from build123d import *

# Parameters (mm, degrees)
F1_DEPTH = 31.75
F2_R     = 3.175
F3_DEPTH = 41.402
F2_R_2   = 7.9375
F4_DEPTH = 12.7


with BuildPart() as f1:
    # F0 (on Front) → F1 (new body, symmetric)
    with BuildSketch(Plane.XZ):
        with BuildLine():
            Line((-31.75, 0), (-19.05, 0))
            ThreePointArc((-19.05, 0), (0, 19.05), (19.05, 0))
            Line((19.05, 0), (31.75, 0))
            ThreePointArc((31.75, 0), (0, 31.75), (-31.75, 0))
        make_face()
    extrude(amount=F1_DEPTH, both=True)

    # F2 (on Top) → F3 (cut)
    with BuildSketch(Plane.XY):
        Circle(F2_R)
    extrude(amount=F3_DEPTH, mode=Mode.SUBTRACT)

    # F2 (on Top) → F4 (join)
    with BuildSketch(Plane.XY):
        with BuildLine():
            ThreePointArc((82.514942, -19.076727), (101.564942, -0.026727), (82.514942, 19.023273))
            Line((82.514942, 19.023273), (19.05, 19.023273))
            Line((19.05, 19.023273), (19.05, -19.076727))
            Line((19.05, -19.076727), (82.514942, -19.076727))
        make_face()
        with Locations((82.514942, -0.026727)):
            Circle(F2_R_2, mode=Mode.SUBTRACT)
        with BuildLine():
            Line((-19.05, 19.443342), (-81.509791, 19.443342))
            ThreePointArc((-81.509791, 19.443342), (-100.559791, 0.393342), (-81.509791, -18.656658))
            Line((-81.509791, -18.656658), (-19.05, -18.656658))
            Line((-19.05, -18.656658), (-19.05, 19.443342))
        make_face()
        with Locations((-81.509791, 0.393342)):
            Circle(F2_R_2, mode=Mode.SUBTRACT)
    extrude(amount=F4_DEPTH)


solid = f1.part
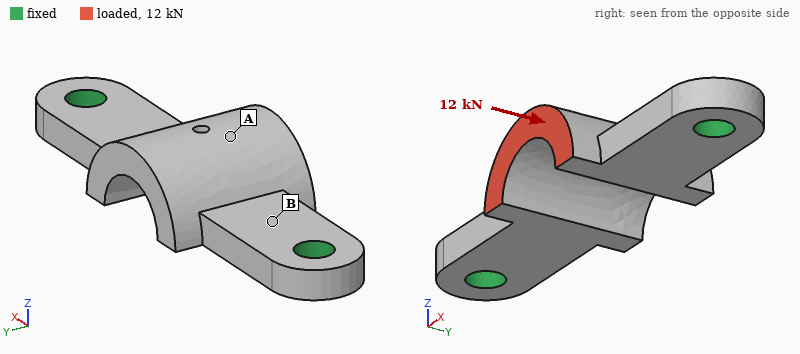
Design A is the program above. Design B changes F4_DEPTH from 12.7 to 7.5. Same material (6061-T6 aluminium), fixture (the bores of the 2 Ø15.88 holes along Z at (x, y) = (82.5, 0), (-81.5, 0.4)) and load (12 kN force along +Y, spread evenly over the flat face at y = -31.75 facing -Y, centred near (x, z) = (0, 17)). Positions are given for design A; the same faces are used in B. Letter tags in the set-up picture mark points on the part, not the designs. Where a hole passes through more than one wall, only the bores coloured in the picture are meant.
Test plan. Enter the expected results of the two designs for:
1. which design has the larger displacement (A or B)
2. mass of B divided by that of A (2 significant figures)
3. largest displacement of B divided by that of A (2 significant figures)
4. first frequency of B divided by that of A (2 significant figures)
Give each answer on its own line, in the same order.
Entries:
B
0.80
3.6
0.52
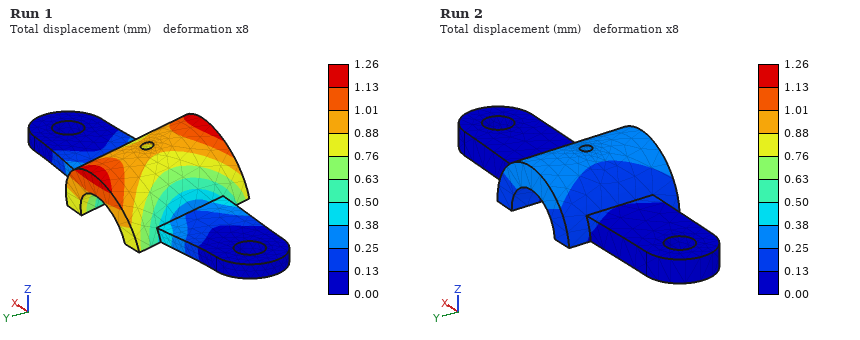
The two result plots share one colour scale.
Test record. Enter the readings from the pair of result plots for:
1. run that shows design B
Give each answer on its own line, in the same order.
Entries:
Run 1
